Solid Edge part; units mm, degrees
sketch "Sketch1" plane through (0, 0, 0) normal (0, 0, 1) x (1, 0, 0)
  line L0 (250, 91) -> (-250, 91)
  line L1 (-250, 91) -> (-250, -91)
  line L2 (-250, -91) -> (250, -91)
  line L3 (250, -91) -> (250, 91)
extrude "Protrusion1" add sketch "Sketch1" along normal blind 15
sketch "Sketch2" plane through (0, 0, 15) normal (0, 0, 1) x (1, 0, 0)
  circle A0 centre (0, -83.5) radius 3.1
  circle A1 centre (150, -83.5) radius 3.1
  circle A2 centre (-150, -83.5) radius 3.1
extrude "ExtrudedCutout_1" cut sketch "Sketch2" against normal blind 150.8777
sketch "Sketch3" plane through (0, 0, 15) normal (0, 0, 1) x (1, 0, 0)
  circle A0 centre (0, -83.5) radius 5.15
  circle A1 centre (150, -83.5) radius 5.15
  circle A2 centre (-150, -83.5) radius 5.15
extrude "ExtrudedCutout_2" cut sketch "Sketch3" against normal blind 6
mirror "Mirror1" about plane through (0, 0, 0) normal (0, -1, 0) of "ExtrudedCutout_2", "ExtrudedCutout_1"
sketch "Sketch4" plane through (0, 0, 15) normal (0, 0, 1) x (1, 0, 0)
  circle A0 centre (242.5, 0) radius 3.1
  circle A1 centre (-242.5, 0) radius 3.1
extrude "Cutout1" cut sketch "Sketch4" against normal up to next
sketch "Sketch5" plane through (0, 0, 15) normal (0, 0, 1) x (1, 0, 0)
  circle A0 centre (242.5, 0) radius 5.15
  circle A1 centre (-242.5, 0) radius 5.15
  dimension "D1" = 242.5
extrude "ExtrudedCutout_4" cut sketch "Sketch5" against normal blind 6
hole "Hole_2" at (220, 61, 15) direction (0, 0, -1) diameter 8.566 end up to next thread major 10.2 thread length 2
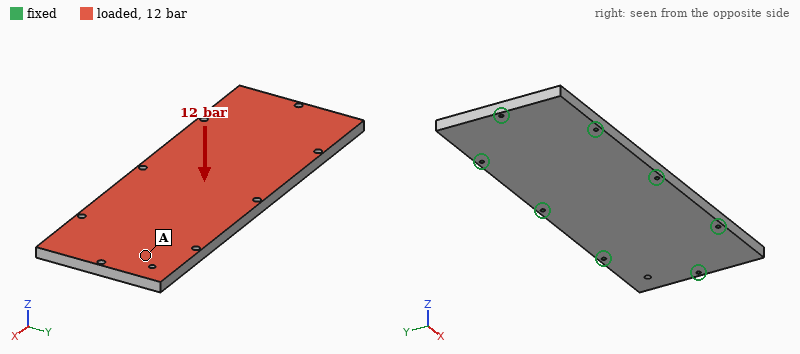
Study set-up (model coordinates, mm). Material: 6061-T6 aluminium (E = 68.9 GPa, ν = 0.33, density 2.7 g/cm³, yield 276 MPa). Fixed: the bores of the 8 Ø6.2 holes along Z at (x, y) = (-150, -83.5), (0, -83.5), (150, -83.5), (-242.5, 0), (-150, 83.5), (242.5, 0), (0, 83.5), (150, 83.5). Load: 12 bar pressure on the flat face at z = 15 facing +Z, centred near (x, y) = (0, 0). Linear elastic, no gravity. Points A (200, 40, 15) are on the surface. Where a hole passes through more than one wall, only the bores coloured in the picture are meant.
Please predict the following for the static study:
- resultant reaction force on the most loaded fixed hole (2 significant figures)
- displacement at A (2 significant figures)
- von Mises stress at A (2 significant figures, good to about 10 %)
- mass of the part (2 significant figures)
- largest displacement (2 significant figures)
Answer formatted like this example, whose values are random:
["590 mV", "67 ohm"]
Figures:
["20 kN", "0.13 mm", "48 MPa", "3.7 kg", "0.43 mm"]
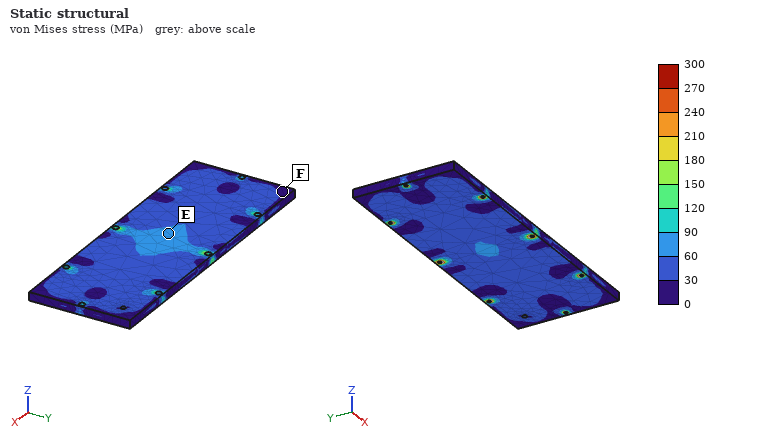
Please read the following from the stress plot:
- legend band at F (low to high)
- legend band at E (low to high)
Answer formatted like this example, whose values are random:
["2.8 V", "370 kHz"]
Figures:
["0 to 30 MPa", "60 to 90 MPa"]
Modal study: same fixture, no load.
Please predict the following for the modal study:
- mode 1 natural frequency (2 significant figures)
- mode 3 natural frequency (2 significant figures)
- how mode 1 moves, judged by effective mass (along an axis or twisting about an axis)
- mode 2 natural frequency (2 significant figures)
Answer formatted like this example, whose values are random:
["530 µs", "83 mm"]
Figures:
["1500 Hz", "1900 Hz", "along Z", "1700 Hz"]
